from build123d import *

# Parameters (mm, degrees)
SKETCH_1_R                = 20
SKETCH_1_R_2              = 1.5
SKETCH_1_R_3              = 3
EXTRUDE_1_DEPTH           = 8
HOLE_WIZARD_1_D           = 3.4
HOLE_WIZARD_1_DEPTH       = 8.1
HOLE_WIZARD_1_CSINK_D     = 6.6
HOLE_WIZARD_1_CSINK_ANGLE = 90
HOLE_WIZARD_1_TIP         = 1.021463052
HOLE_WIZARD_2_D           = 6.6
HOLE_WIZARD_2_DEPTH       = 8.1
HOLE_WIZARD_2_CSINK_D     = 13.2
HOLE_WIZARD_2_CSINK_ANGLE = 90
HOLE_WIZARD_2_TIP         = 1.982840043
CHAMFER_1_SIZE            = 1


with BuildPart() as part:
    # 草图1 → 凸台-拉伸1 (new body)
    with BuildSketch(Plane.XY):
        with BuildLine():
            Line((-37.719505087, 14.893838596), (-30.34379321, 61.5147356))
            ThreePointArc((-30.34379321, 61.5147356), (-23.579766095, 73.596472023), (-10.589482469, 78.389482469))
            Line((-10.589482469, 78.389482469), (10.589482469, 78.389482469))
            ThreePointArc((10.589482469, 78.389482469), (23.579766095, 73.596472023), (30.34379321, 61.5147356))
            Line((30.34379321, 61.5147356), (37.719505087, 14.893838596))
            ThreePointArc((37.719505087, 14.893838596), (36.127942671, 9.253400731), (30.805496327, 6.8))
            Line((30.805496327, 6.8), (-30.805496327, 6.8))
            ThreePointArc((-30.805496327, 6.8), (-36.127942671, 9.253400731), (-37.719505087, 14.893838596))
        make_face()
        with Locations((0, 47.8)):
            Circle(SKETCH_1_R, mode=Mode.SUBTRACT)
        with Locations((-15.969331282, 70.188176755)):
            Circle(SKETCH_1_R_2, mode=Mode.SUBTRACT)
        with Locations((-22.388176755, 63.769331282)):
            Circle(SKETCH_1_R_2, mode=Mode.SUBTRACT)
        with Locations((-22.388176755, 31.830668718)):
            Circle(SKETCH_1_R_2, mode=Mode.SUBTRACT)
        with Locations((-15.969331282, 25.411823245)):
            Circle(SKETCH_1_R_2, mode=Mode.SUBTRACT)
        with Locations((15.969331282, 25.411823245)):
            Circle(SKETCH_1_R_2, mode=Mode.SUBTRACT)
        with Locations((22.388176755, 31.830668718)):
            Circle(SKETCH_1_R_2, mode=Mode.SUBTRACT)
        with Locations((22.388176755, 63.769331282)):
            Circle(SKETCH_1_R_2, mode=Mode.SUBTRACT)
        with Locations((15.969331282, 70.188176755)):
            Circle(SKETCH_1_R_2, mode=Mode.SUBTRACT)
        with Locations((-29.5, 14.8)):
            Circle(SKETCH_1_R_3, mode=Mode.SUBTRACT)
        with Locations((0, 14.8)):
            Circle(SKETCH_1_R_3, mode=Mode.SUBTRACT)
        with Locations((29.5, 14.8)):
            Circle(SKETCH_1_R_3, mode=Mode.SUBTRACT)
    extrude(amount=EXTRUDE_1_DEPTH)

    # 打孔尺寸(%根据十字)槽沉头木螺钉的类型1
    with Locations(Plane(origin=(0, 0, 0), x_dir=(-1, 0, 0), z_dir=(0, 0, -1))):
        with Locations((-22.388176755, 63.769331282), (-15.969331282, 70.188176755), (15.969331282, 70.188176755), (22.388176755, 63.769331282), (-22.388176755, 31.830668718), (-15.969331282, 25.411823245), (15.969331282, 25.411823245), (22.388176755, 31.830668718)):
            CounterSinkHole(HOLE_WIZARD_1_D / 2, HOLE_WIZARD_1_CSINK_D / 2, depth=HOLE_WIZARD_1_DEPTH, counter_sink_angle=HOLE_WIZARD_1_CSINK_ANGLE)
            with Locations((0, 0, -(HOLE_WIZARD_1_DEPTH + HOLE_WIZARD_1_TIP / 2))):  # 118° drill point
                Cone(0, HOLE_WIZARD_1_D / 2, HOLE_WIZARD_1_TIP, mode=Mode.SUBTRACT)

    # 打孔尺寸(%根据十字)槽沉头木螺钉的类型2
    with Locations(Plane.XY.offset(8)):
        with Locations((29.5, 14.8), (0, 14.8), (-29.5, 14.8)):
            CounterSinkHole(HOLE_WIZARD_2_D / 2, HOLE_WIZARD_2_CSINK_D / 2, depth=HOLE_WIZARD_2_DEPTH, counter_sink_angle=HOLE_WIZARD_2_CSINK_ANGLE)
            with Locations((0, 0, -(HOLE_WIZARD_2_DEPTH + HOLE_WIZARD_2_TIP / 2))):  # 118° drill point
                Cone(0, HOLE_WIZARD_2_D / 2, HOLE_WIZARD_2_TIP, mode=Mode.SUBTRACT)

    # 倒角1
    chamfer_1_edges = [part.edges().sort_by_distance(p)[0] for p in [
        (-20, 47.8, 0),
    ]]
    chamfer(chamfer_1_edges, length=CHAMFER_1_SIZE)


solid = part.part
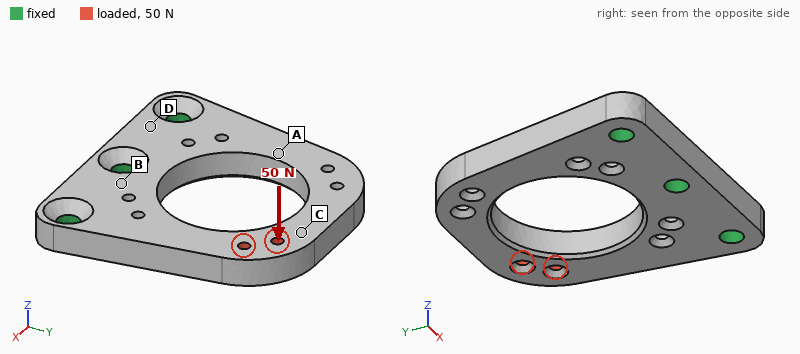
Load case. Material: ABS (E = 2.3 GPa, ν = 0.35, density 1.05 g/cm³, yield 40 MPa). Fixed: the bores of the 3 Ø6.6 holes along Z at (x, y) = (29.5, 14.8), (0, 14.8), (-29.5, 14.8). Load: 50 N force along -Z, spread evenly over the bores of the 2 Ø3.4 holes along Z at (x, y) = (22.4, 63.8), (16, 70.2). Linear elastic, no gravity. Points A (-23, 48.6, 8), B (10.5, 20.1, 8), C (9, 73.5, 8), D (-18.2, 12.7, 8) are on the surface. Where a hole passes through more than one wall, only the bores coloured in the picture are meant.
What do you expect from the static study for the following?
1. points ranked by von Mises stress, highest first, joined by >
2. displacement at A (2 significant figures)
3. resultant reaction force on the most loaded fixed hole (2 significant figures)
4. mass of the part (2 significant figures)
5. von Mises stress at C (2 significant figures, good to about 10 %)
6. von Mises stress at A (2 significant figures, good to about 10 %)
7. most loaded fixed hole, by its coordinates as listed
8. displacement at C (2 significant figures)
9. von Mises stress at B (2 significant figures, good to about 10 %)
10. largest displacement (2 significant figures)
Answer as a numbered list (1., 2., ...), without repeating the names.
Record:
1. A > B > C > D
2. 0.25 mm
3. 34 N
4. 26 g
5. 1.7 MPa
6. 4.0 MPa
7. (29.5, 14.8)
8. 0.94 mm
9. 2.8 MPa
10. 1.1 mm
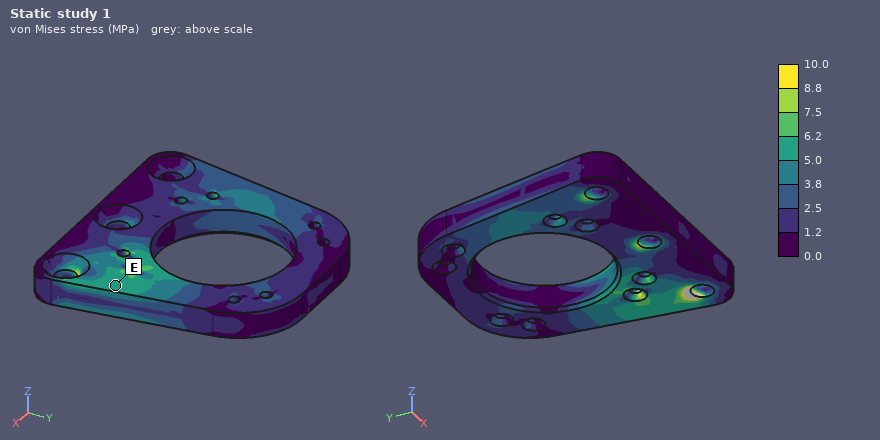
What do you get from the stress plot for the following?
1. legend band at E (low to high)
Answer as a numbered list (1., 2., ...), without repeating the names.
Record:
1. 5.0 to 6.2 MPa
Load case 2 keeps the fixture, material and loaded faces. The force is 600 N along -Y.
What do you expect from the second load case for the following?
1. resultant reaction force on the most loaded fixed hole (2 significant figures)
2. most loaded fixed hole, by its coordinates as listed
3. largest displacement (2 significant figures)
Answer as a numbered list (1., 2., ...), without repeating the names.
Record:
1. 480 N
2. (29.5, 14.8)
3. 0.45 mm
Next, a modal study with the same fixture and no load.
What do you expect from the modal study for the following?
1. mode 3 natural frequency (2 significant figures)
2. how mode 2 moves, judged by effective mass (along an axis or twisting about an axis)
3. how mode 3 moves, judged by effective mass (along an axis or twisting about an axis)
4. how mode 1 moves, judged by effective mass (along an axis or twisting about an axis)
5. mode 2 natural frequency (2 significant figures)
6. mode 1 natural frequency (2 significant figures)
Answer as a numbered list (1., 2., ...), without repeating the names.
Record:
1. 1900 Hz
2. twisting about Y
3. along X
4. along Z
5. 1100 Hz
6. 450 Hz
